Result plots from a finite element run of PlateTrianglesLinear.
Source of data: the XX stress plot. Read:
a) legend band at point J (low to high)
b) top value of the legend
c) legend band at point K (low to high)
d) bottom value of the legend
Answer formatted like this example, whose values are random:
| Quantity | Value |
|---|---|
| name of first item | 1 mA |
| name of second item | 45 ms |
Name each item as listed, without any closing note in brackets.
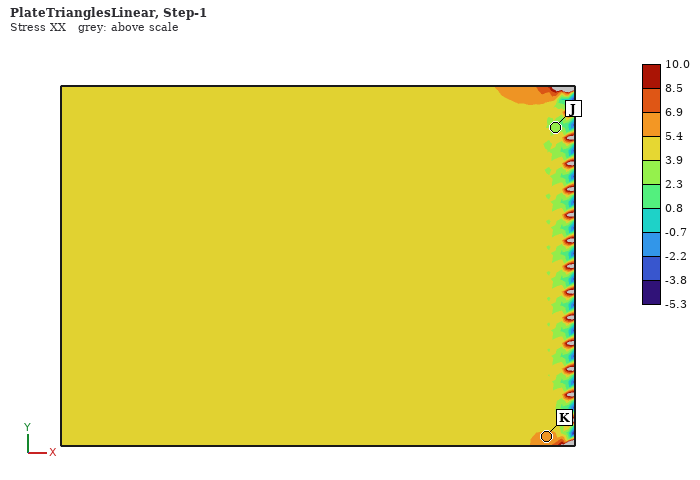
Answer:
| Quantity | Value |
|---|---|
| legend band at point J | 2.3 to 3.9 |
| top value of the legend | 10.0 |
| legend band at point K | 5.4 to 6.9 |
| bottom value of the legend | -5.3 |
